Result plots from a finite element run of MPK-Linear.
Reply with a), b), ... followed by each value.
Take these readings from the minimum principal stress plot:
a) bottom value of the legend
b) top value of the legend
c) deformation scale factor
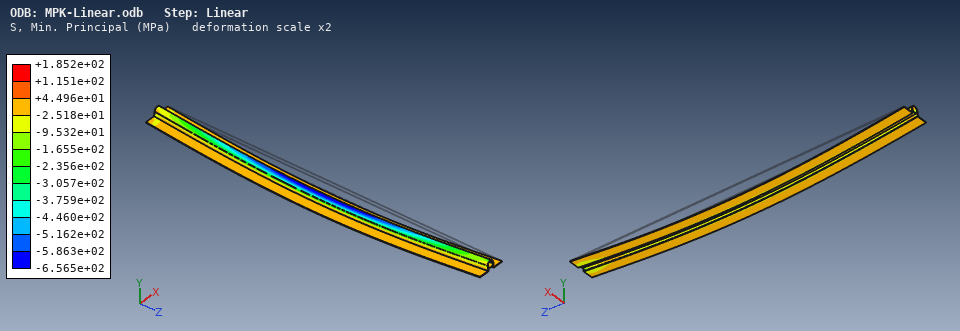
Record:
a) -6.565e+02 MPa
b) +1.852e+02 MPa
c) 2
